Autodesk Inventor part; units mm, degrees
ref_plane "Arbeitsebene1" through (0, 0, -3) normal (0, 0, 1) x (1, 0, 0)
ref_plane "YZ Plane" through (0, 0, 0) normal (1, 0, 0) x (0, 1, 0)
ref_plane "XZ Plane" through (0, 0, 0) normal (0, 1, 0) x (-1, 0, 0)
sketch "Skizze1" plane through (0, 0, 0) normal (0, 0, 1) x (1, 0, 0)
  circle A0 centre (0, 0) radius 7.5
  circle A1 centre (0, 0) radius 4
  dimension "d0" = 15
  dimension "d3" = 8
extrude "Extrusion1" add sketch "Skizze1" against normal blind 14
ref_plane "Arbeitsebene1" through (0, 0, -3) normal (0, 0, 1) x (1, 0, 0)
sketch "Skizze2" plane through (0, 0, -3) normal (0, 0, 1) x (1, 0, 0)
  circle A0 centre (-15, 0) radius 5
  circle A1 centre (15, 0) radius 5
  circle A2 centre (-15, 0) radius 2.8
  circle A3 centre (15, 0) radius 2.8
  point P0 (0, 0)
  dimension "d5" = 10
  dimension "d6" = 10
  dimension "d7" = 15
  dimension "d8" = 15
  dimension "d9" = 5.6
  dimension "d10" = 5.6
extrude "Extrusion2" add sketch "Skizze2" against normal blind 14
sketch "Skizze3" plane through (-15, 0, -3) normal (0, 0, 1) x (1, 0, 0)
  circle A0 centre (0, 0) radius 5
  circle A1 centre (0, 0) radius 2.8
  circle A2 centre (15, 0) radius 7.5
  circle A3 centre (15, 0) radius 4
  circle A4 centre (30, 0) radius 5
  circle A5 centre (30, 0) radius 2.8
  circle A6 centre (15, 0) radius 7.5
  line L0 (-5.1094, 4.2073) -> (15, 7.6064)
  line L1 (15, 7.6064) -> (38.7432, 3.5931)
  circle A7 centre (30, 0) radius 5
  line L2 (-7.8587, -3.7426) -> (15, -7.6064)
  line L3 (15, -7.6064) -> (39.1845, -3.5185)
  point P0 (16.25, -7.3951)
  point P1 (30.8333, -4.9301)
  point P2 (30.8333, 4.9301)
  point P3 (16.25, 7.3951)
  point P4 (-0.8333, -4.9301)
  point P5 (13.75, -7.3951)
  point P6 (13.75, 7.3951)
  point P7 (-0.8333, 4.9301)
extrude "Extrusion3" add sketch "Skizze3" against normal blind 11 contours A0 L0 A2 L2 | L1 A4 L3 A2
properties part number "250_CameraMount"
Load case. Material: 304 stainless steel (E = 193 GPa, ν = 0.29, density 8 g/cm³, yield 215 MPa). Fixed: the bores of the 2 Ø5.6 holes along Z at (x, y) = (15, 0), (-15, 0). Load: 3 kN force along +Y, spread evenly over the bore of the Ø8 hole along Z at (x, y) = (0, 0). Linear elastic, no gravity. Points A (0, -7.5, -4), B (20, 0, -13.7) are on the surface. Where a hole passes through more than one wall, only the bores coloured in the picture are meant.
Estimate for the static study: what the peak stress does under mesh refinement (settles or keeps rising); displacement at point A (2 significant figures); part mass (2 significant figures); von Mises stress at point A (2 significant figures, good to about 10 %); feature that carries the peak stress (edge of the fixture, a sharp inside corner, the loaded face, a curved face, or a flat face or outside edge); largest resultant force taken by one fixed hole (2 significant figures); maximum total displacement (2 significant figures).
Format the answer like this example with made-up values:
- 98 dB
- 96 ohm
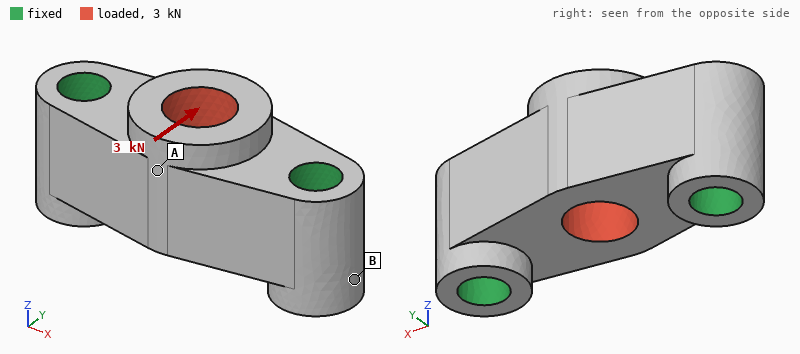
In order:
- keeps rising
- 3.3 µm
- 37 g
- 24 MPa
- edge of the fixture
- 1.5 kN
- 3.9 µm
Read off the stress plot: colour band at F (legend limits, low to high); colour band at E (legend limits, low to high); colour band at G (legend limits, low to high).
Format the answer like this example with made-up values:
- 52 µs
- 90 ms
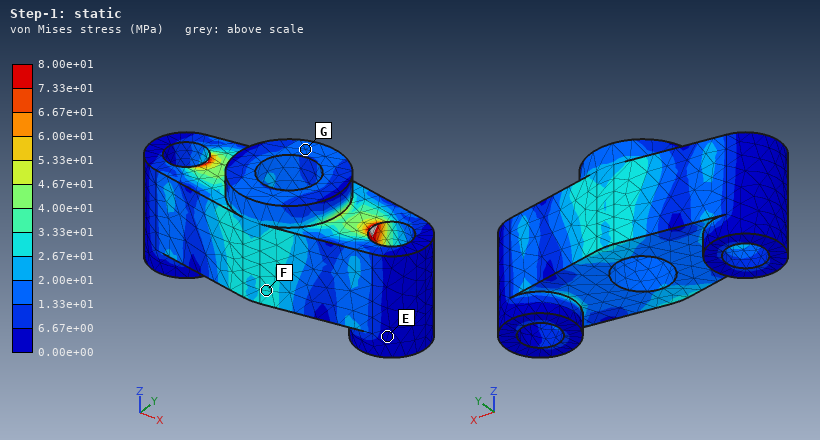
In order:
- 2.67e+01 to 3.33e+01 MPa
- 0.00e+00 to 6.67e+00 MPa
- 1.33e+01 to 2.00e+01 MPa
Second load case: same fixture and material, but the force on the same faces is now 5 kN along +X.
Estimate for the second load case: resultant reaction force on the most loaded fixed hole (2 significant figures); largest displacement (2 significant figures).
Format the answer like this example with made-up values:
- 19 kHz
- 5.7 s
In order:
- 2.5 kN
- 1.9 µm
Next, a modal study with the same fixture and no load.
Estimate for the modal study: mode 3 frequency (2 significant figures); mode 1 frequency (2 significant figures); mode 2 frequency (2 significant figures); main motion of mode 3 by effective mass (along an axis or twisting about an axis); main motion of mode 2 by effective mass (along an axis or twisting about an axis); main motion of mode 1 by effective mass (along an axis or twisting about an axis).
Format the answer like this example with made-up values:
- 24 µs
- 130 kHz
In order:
- 48 kHz
- 38 kHz
- 44 kHz
- along Y
- along Z
- along Y
